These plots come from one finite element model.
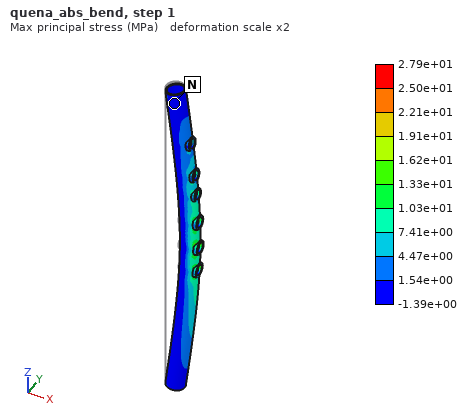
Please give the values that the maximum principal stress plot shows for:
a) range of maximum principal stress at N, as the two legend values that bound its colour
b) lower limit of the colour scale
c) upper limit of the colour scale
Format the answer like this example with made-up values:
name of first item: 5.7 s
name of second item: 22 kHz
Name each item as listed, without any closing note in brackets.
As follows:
range of maximum principal stress at N, as the two legend values that bound its colour: -1.39e+00 to 1.54e+00 MPa
lower limit of the colour scale: -1.39e+00 MPa
upper limit of the colour scale: 2.79e+01 MPa
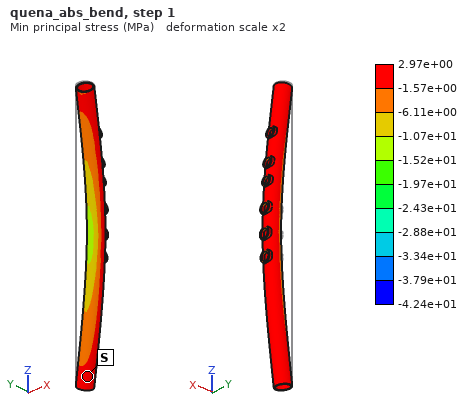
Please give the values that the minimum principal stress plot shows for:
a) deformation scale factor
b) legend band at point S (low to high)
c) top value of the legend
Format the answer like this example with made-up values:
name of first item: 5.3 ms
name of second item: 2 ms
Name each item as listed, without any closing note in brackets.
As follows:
deformation scale factor: 2
legend band at point S: -1.57e+00 to 2.97e+00 MPa
top value of the legend: 2.97e+00 MPa
